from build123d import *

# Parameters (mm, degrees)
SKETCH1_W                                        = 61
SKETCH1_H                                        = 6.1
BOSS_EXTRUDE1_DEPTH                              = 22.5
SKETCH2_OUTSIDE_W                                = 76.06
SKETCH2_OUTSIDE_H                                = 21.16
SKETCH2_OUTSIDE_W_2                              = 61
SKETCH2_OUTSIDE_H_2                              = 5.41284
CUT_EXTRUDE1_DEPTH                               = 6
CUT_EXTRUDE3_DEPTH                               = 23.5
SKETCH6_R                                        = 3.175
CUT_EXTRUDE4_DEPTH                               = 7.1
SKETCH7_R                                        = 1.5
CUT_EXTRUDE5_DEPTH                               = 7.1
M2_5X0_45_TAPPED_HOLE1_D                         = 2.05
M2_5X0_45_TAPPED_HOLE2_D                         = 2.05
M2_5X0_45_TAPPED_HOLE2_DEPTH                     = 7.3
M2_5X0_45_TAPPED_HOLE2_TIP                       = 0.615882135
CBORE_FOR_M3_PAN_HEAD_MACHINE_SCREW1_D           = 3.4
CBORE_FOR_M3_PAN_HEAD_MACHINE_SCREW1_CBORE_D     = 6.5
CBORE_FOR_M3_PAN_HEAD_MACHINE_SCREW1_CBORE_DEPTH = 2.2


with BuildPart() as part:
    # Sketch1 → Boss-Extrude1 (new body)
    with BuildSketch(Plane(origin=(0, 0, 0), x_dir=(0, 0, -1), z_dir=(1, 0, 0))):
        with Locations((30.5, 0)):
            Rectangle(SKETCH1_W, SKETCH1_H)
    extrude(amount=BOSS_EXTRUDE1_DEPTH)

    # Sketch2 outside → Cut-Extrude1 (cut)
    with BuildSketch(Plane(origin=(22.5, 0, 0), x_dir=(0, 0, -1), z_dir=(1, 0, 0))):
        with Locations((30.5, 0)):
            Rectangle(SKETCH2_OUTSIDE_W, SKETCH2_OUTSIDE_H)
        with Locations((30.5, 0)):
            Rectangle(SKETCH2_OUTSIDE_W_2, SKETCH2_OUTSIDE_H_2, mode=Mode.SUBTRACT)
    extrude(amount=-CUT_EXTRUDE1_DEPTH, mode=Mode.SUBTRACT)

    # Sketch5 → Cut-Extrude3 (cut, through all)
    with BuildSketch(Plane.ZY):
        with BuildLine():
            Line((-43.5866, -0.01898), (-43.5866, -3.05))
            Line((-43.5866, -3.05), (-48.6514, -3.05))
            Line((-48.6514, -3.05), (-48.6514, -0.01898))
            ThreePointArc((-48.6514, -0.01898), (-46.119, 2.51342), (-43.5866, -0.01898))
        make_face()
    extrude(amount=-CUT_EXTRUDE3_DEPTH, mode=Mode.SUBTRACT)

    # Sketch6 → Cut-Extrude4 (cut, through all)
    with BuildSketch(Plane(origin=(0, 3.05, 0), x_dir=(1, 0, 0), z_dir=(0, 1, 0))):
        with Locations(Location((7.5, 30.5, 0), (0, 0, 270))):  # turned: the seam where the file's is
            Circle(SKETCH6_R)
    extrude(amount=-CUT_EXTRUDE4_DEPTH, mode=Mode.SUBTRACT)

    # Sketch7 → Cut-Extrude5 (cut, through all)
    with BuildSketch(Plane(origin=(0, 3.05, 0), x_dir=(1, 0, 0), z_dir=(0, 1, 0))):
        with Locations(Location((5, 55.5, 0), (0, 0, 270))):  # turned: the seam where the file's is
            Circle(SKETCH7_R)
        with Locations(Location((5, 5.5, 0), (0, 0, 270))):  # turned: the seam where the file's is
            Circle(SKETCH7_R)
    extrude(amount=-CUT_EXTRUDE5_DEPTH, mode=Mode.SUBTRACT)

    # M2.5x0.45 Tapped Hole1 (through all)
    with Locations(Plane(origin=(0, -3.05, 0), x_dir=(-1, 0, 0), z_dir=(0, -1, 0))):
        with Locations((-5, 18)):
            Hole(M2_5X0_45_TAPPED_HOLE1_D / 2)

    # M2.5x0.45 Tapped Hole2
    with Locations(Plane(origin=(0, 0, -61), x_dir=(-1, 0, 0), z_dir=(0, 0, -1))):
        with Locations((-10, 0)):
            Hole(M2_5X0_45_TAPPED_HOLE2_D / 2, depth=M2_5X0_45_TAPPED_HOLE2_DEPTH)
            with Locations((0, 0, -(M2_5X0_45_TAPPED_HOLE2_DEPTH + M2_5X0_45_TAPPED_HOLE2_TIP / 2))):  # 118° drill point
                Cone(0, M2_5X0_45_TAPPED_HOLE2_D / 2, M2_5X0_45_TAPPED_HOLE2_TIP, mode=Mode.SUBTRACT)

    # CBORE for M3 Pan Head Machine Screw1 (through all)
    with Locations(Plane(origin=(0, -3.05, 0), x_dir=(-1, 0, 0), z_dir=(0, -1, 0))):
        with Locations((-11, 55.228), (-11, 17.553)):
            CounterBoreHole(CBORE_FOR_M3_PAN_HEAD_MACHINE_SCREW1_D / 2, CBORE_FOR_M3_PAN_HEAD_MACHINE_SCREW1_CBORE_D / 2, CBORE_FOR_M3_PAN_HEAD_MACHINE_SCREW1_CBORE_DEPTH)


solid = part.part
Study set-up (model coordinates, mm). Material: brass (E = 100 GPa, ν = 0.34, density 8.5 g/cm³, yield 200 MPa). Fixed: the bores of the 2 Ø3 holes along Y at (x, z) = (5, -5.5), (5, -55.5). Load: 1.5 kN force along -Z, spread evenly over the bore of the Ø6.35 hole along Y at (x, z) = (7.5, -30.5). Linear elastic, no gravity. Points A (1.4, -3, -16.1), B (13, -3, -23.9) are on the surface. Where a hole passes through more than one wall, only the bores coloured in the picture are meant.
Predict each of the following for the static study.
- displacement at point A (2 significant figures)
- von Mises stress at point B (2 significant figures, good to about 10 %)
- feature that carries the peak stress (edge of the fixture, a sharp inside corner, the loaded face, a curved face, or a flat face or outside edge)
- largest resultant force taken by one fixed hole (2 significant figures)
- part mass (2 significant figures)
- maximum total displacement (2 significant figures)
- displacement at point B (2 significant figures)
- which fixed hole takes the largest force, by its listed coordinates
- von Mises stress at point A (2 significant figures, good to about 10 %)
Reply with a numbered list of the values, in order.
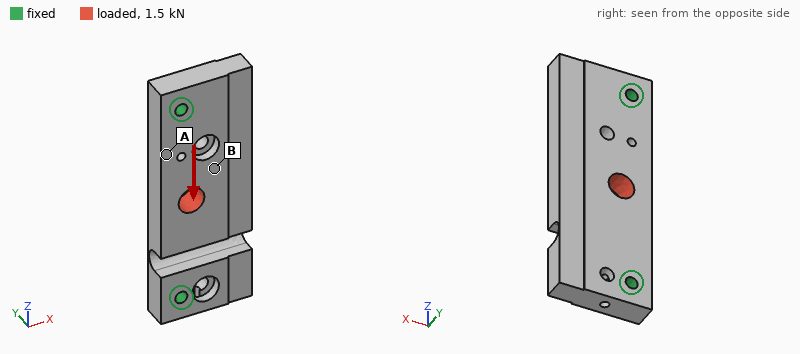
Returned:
1. 1.9 µm
2. 10 MPa
3. a curved face
4. 1.2 kN
5. 60 g
6. 7.0 µm
7. 4.5 µm
8. (5, -5.5)
9. 22 MPa
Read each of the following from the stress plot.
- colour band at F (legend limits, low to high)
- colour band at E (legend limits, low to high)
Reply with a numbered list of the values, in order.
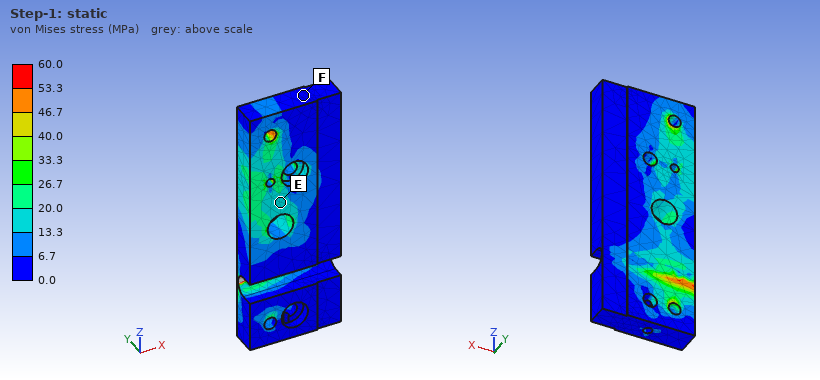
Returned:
1. 0.0 to 6.7 MPa
2. 13.3 to 20.0 MPa
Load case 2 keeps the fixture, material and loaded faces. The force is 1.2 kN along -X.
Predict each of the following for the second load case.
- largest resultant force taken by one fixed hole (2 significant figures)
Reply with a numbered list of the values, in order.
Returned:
1. 670 N
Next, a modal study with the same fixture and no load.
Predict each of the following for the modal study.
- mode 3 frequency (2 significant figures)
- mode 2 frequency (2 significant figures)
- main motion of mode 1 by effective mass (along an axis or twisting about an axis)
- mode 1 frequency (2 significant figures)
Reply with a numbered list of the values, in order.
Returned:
1. 8400 Hz
2. 6300 Hz
3. along Y
4. 4200 Hz
